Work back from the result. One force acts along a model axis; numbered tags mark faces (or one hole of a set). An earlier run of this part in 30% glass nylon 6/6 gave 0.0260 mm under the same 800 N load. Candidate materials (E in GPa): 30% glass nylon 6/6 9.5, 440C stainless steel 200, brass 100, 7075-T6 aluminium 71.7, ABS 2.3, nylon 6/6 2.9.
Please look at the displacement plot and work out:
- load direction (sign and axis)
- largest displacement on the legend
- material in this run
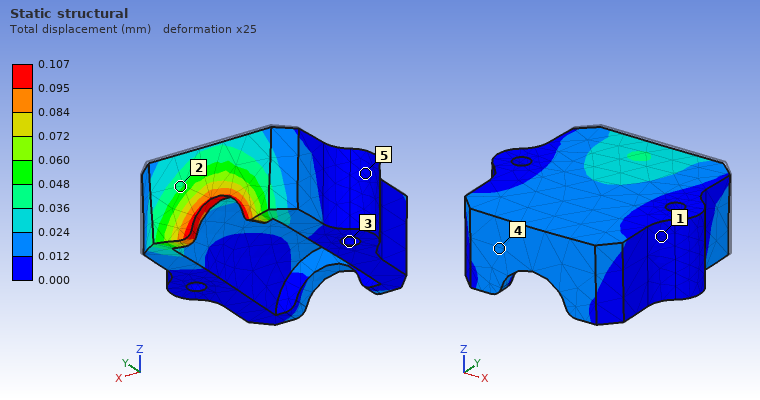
-Y
0.107 mm
ABS
